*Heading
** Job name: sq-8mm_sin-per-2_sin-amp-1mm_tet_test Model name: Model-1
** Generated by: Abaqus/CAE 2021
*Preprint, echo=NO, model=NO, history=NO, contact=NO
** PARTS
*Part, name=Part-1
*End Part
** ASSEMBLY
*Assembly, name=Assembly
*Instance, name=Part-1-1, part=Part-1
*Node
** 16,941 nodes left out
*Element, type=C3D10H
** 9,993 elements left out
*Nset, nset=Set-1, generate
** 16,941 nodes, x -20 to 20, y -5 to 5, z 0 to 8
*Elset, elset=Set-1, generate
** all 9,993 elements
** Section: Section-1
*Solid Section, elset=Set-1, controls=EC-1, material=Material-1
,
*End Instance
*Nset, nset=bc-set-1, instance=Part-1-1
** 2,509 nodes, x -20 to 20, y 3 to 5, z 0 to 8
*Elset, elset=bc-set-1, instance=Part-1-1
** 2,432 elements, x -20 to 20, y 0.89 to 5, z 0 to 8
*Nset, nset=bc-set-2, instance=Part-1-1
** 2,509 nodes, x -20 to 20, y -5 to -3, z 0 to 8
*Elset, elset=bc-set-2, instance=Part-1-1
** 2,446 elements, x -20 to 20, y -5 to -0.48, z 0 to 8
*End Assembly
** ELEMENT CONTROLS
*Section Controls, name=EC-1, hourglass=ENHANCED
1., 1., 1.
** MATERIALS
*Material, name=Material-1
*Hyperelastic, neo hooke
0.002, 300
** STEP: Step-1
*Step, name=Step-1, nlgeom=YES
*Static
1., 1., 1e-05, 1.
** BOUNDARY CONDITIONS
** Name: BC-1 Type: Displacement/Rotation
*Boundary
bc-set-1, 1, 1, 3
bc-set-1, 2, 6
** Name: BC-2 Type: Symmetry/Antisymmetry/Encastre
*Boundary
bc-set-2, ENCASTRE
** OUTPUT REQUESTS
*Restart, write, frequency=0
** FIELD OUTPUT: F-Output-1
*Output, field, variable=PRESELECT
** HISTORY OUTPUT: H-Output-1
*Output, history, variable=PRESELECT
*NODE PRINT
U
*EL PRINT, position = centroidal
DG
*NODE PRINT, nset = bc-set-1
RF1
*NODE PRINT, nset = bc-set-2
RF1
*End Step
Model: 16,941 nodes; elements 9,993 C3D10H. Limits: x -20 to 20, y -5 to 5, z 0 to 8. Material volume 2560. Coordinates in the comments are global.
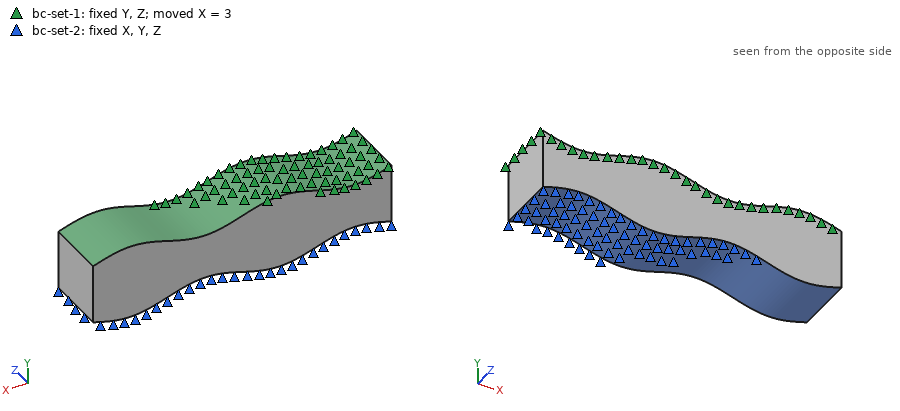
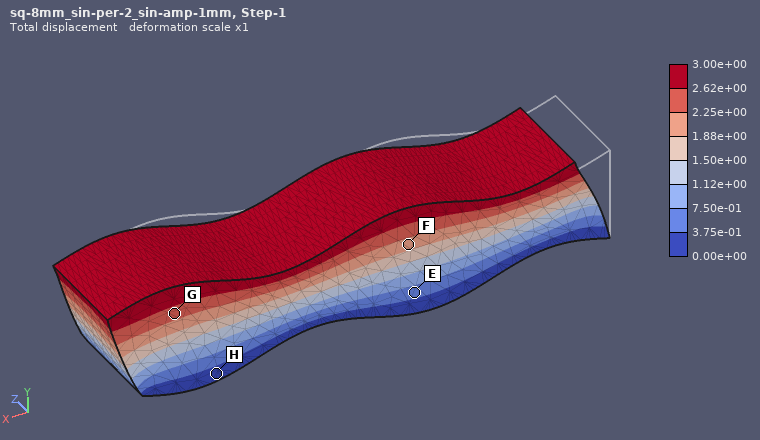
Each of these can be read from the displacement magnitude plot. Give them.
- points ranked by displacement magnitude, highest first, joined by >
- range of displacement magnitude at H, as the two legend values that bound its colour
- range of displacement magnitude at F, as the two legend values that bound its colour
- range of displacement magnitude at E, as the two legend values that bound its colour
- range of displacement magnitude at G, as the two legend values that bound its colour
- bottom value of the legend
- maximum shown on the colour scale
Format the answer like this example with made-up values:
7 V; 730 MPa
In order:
G > F > E > H; 0.00e+00 to 3.75e-01; 1.88e+00 to 2.25e+00; 3.75e-01 to 7.50e-01; 2.25e+00 to 2.62e+00; 0.00e+00; 3.00e+00
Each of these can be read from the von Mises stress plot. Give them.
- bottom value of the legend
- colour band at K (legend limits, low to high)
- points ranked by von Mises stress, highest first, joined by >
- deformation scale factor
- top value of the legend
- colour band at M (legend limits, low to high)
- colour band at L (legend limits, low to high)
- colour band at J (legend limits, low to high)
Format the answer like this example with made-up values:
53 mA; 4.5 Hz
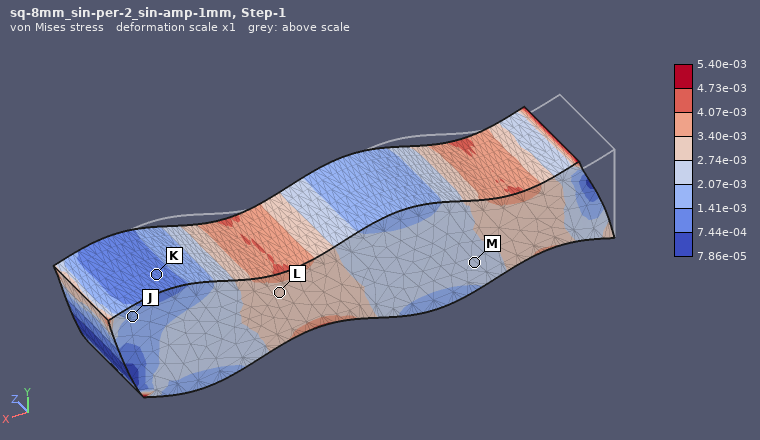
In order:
7.86e-05; 7.44e-04 to 1.41e-03; L > M > J > K; 1; 5.40e-03; 2.07e-03 to 2.74e-03; 2.74e-03 to 3.40e-03; 1.41e-03 to 2.07e-03
